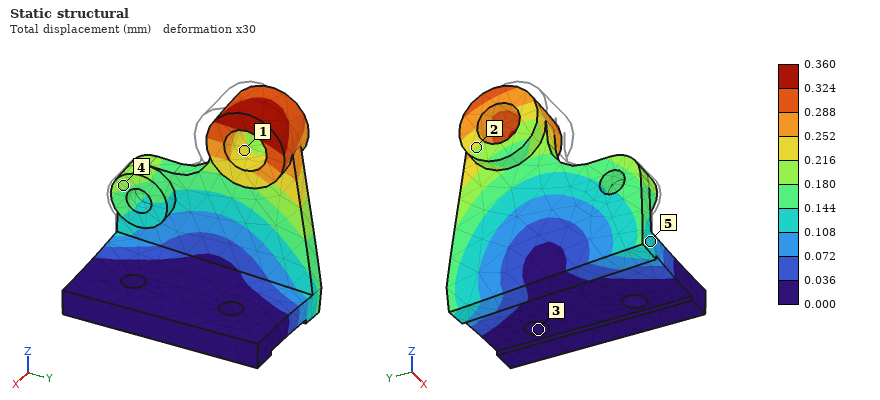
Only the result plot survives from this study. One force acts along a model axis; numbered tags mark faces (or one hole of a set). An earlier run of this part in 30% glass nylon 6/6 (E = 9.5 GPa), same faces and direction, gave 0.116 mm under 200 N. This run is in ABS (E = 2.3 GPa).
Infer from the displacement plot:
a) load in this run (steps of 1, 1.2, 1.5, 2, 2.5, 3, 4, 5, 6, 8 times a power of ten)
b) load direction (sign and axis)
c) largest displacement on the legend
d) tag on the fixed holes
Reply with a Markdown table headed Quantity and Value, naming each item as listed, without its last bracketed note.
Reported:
| Quantity | Value |
|---|---|
| load in this run | 150 N |
| load direction | +Y |
| largest displacement on the legend | 0.360 mm |
| tag on the fixed holes | 3 |
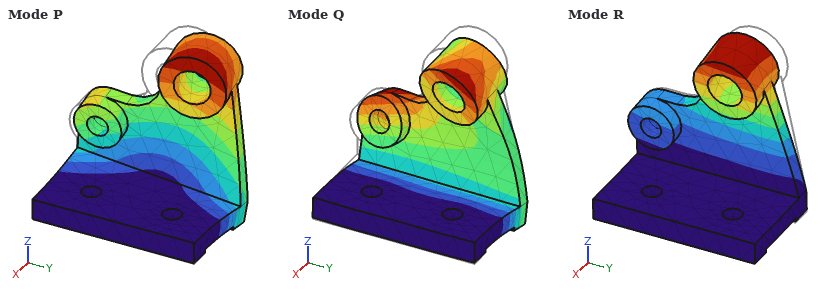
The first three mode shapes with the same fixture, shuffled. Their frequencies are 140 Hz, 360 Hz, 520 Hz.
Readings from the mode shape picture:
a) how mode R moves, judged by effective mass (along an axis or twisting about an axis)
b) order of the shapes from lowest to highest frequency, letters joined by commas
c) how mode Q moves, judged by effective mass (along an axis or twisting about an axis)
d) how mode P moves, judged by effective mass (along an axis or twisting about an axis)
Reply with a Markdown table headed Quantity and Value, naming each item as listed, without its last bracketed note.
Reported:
| Quantity | Value |
|---|---|
| how mode R moves, judged by effective mass | along X |
| order of the shapes from lowest to highest frequency, letters joined by commas | R, P, Q |
| how mode Q moves, judged by effective mass | along Z |
| how mode P moves, judged by effective mass | along Y |
